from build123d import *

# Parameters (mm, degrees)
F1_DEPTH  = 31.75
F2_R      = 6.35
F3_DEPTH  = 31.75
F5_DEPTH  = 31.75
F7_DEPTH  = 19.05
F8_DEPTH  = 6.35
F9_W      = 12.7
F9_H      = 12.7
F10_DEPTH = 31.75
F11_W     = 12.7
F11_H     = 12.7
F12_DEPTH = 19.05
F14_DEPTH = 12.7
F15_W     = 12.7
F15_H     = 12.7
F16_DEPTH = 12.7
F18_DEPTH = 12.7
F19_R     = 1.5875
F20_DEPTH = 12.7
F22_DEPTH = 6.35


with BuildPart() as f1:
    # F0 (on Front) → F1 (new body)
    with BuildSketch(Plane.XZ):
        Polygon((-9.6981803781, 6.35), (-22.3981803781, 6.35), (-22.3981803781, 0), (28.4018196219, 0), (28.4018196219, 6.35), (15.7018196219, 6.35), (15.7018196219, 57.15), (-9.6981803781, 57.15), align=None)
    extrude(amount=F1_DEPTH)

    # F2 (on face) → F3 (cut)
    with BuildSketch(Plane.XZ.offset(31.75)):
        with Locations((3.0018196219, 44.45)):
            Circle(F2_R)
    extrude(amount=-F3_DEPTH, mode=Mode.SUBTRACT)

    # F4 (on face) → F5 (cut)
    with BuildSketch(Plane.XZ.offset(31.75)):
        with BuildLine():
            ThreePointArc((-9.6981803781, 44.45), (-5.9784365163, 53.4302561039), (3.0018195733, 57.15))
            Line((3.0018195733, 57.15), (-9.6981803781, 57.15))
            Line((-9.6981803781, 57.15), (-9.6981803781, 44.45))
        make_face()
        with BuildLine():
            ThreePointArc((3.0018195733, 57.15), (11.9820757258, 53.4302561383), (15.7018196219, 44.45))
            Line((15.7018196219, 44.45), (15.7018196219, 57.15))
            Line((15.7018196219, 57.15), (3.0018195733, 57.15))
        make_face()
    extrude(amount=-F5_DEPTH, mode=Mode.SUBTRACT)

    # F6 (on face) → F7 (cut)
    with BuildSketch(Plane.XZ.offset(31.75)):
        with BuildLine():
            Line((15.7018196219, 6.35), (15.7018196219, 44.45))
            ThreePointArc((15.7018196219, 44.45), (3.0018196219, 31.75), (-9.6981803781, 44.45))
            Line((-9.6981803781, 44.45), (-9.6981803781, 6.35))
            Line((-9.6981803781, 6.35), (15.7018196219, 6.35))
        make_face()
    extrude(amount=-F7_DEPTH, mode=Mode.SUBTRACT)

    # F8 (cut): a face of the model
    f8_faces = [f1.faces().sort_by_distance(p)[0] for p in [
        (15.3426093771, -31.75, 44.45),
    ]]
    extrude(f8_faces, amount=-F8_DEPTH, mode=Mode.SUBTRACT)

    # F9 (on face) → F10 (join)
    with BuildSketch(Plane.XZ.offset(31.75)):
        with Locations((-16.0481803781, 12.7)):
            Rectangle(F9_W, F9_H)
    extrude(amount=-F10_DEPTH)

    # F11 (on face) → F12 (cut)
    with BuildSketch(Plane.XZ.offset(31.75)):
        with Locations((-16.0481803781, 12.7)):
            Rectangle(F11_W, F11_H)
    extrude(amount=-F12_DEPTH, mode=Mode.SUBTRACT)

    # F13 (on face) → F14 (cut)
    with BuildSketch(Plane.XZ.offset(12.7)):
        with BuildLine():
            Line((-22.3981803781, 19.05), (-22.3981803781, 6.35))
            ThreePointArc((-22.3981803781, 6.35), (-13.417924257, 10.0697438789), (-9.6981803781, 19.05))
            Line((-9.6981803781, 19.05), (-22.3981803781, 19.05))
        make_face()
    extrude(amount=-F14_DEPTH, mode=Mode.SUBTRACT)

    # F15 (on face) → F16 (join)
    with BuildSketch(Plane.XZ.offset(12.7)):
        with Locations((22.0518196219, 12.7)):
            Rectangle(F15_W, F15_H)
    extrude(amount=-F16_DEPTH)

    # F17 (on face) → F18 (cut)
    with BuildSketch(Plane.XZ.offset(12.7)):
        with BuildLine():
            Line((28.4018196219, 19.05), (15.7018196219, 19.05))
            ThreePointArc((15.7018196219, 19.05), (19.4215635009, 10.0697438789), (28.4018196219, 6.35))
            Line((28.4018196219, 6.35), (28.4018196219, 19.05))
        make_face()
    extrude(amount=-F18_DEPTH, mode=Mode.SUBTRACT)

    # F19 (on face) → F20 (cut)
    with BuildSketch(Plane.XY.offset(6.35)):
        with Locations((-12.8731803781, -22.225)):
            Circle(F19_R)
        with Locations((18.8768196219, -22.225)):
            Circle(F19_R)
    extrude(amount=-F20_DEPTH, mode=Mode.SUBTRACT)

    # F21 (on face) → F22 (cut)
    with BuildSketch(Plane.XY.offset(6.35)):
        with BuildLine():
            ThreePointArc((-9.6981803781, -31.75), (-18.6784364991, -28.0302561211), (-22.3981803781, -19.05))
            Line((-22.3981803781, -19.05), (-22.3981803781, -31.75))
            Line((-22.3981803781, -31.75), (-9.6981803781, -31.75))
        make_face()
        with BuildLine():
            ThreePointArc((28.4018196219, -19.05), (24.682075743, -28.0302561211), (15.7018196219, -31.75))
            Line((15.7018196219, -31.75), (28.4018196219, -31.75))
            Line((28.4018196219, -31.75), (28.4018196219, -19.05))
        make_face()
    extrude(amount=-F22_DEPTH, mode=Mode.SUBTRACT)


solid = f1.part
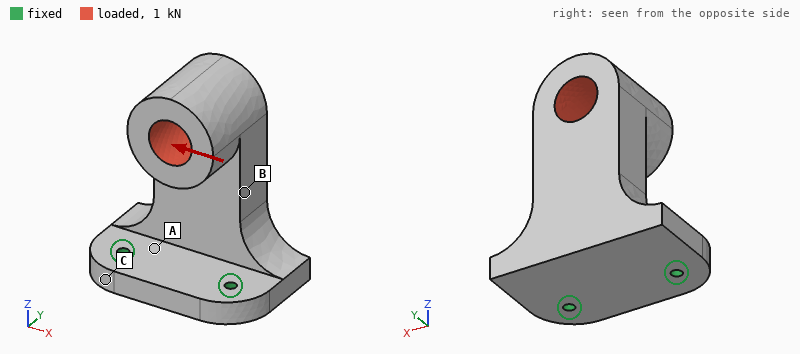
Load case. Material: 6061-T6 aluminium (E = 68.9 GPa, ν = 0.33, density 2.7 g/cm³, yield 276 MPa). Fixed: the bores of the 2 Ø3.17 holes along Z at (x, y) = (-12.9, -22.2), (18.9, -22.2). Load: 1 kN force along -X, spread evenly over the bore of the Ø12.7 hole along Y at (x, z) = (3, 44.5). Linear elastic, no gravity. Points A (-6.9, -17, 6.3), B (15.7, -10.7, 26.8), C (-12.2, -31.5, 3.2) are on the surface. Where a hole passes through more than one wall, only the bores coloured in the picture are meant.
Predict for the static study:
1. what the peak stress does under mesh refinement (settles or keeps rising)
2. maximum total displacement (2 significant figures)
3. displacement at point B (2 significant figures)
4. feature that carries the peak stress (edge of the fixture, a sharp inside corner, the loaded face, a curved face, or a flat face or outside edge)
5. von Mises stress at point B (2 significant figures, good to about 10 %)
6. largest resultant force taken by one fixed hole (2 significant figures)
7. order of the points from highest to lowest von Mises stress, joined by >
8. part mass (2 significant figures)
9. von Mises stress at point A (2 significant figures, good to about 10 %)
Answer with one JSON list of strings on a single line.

["keeps rising", "0.12 mm", "0.049 mm", "edge of the fixture", "17 MPa", "1.3 kN", "A > B > C", "79 g", "33 MPa"]
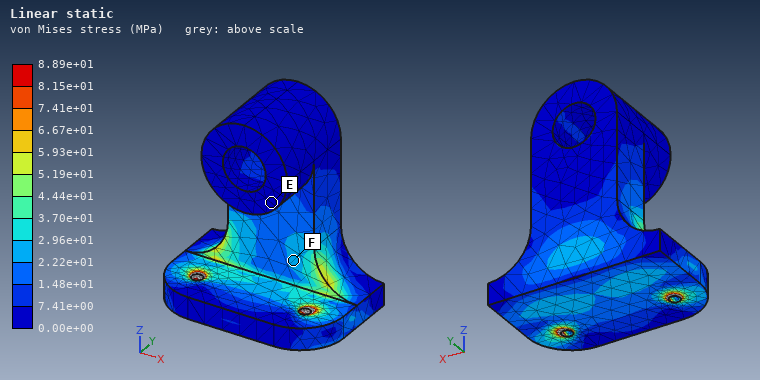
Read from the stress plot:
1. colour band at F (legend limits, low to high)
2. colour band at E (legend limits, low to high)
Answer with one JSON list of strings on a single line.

["2.22e+01 to 2.96e+01 MPa", "0.00e+00 to 7.41e+00 MPa"]
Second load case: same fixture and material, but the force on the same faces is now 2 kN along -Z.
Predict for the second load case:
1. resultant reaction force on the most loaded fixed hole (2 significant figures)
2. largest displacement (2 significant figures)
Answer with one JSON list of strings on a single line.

["1.0 kN", "67 µm"]
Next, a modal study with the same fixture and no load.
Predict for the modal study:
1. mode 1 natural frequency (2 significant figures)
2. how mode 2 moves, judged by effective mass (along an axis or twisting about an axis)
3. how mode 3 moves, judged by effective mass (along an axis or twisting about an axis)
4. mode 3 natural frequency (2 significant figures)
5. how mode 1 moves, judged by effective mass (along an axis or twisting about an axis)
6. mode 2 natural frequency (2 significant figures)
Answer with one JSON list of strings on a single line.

["1300 Hz", "along X", "along Z", "5700 Hz", "along Y", "3100 Hz"]
